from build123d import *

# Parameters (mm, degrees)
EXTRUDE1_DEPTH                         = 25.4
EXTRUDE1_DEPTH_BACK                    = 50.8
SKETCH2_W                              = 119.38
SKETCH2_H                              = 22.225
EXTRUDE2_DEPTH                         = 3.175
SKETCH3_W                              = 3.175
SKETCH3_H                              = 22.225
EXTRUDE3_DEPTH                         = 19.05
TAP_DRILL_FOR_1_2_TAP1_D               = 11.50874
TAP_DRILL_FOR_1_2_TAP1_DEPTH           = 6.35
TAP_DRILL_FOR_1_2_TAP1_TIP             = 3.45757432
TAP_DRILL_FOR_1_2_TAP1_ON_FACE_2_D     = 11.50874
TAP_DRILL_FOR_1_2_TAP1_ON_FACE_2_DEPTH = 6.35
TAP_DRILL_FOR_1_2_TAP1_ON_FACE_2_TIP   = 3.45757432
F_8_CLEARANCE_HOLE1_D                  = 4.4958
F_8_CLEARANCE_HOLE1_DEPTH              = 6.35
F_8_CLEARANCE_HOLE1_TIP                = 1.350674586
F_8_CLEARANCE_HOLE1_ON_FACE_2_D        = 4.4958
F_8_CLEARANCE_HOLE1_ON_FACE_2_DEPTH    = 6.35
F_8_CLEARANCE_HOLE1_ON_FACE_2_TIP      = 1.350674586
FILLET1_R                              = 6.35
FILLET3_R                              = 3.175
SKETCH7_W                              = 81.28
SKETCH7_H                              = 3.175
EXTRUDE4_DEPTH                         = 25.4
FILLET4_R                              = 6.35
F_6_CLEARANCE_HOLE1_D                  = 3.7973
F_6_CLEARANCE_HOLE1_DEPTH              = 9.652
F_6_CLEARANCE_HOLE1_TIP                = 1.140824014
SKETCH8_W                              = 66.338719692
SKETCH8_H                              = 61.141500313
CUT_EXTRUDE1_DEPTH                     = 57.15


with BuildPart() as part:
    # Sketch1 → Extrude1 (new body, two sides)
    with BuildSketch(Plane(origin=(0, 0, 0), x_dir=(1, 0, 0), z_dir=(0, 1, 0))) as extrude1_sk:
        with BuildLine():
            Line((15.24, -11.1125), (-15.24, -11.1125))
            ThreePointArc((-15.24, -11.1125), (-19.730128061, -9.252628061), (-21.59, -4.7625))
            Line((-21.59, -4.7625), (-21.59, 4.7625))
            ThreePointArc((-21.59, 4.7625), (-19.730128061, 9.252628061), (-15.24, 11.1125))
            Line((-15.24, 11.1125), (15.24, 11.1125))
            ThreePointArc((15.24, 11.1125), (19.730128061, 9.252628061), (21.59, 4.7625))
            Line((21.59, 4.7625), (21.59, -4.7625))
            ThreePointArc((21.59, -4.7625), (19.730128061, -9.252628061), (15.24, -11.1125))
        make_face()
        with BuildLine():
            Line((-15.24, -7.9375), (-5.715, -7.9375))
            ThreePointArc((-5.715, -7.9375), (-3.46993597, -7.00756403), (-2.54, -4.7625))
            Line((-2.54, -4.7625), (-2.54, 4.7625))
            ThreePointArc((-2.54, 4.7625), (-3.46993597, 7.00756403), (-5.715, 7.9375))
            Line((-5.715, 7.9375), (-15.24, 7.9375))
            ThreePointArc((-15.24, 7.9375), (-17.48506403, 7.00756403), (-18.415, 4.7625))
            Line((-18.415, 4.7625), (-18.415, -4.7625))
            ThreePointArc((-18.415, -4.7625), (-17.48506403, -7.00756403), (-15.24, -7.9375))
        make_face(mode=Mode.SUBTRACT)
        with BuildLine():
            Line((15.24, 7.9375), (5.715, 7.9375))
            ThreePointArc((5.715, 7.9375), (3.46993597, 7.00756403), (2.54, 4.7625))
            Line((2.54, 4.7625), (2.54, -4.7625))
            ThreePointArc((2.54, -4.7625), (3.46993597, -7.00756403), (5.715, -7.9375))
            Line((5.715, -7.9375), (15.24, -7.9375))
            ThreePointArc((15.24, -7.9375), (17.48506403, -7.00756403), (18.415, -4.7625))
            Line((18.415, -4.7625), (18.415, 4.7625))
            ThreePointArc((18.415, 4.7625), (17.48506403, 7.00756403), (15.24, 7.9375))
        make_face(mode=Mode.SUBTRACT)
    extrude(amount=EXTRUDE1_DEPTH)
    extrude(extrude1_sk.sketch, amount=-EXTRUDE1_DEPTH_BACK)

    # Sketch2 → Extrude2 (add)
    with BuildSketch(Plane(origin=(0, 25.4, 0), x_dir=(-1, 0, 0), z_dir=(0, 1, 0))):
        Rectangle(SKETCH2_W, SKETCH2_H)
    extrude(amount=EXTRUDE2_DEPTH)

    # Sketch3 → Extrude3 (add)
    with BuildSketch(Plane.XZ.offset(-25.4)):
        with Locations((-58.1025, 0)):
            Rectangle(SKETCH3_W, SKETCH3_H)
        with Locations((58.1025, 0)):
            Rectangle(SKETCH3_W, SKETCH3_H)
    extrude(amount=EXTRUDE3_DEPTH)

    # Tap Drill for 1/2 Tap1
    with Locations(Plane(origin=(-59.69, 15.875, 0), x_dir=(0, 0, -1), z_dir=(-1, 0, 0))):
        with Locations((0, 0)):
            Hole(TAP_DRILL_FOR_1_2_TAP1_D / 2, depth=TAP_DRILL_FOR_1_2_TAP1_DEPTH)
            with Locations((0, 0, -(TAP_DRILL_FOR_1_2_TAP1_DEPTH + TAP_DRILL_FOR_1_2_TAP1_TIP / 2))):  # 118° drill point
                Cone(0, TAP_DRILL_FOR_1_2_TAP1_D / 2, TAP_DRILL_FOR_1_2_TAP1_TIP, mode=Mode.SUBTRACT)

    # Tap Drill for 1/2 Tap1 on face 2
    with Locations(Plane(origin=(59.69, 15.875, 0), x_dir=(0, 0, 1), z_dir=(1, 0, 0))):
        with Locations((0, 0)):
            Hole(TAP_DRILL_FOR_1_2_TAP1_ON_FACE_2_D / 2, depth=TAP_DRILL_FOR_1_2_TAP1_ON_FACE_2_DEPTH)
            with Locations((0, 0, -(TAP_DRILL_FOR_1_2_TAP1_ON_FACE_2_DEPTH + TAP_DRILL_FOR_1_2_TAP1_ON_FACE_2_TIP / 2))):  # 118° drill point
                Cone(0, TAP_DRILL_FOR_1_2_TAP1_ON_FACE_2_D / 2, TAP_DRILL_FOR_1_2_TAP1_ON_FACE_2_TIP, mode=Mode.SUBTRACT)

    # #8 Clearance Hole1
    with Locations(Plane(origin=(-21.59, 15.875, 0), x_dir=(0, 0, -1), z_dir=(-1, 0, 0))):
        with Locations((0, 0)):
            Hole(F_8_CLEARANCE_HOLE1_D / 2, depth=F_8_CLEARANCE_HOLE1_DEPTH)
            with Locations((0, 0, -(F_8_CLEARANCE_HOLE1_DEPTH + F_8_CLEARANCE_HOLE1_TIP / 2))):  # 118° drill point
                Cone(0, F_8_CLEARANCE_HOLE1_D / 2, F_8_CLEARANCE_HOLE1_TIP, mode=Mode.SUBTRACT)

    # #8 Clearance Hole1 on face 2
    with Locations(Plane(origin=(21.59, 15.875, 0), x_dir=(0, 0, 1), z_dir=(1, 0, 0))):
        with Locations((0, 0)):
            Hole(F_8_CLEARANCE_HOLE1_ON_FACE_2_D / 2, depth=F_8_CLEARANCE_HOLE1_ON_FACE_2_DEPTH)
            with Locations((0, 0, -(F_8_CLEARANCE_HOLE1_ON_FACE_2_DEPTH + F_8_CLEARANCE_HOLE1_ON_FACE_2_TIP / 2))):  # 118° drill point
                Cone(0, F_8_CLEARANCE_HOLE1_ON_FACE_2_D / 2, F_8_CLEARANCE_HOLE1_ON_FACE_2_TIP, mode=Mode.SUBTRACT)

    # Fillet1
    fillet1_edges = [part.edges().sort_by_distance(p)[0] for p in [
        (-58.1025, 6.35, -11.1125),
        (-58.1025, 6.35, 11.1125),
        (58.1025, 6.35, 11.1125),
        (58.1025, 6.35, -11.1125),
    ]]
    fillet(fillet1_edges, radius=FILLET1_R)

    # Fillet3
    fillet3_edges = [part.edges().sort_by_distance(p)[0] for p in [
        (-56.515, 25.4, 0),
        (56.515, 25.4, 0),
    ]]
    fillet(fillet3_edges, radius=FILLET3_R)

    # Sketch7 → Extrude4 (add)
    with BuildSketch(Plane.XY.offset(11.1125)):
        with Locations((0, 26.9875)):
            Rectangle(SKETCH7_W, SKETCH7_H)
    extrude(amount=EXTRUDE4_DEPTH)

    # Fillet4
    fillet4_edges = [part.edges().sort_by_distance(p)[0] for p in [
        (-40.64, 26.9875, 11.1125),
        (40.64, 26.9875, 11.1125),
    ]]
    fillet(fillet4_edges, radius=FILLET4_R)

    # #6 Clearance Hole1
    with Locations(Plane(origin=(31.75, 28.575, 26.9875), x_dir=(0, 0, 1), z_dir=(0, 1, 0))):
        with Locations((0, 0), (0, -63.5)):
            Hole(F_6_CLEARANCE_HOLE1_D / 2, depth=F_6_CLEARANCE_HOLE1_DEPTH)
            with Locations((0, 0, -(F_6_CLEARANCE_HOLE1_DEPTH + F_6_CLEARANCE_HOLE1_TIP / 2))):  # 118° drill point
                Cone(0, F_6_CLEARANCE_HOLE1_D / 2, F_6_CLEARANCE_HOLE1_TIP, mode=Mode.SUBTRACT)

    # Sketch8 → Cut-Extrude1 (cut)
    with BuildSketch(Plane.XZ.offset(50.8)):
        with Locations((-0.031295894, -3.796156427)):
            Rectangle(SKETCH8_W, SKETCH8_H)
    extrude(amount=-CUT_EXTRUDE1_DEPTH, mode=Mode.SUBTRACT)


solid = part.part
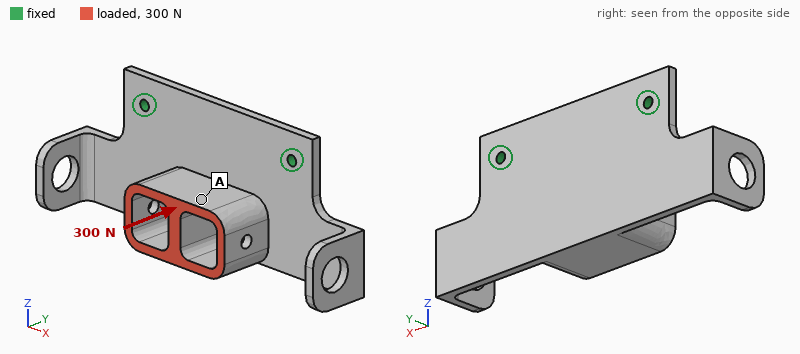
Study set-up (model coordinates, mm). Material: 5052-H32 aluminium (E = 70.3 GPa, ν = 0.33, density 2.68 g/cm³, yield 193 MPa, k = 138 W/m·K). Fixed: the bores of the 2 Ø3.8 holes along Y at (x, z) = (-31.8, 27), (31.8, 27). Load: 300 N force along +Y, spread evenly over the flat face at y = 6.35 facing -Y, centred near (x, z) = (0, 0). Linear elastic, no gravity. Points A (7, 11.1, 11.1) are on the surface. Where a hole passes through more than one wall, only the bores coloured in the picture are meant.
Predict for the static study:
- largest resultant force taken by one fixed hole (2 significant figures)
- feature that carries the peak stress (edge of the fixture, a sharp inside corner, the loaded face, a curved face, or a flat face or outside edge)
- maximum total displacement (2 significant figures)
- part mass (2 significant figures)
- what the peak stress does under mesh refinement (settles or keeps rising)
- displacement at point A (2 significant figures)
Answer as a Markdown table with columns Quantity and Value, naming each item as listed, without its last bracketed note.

| Quantity | Value |
|---|---|
| largest resultant force taken by one fixed hole | 150 N |
| feature that carries the peak stress | edge of the fixture |
| maximum total displacement | 0.36 mm |
| part mass | 68 g |
| what the peak stress does under mesh refinement | keeps rising |
| displacement at point A | 0.18 mm |
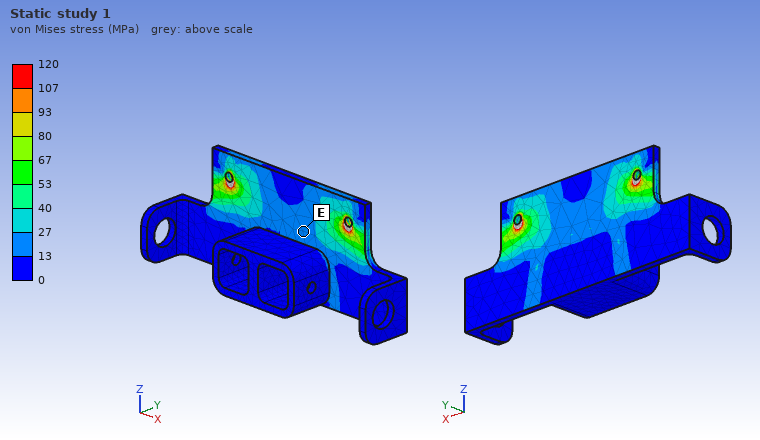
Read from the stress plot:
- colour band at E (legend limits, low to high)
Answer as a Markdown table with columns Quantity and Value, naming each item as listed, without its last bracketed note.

| Quantity | Value |
|---|---|
| colour band at E | 13 to 27 MPa |
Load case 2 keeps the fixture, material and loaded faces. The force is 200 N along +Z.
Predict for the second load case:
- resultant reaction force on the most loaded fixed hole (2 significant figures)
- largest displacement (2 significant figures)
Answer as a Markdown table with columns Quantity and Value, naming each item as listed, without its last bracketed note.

| Quantity | Value |
|---|---|
| resultant reaction force on the most loaded fixed hole | 110 N |
| largest displacement | 0.24 mm |
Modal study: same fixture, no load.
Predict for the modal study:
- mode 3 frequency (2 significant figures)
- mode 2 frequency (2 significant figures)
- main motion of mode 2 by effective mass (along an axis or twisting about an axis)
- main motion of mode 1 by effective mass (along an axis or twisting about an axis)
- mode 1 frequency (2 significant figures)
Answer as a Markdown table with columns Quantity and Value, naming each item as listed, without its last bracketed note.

| Quantity | Value |
|---|---|
| mode 3 frequency | 1400 Hz |
| mode 2 frequency | 1200 Hz |
| main motion of mode 2 by effective mass | twisting about Z |
| main motion of mode 1 by effective mass | along Y |
| mode 1 frequency | 780 Hz |
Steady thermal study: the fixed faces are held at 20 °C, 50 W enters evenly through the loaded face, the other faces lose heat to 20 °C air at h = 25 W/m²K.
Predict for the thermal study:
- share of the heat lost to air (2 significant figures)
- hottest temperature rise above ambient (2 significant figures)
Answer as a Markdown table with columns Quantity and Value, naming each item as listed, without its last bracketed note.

| Quantity | Value |
|---|---|
| share of the heat lost to air | 26 % |
| hottest temperature rise above ambient | 59 K |
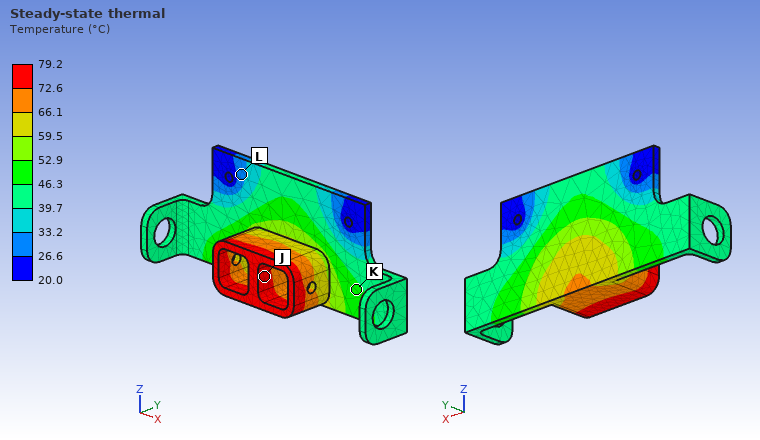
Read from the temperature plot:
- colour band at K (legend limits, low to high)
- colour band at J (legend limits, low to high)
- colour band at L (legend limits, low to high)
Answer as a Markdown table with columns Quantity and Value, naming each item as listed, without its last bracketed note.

| Quantity | Value |
|---|---|
| colour band at K | 46.3 to 52.9 °C |
| colour band at J | 72.6 to 79.2 °C |
| colour band at L | 26.6 to 33.2 °C |
